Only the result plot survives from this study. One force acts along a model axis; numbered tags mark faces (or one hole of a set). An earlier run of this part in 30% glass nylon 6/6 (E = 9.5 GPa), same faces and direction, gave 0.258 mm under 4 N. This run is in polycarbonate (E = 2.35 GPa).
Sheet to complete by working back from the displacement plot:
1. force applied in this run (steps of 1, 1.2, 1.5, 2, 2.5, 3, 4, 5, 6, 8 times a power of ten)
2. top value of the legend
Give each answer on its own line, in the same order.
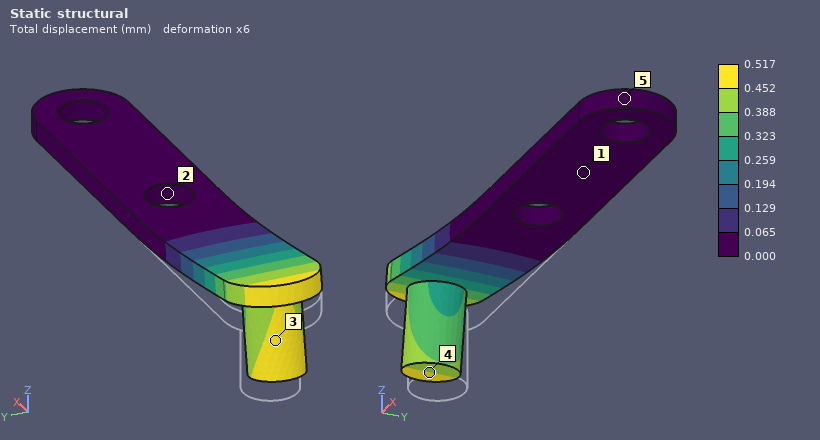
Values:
2 N
0.517 mm
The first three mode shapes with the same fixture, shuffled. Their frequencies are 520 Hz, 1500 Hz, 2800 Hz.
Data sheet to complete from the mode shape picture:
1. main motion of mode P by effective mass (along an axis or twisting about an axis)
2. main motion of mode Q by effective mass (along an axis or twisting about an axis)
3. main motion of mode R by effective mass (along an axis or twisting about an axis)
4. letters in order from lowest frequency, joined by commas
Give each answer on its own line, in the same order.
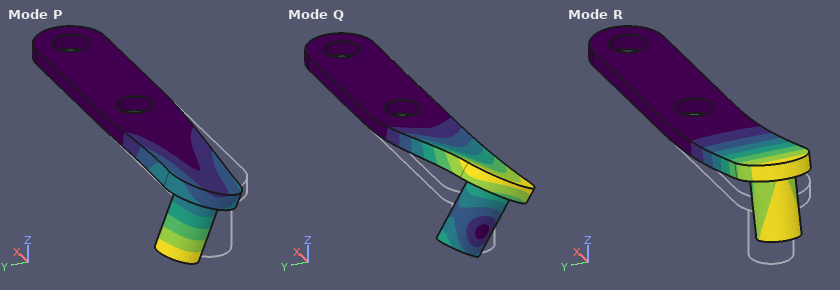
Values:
along Y
along Y
along Z
R, P, Q
